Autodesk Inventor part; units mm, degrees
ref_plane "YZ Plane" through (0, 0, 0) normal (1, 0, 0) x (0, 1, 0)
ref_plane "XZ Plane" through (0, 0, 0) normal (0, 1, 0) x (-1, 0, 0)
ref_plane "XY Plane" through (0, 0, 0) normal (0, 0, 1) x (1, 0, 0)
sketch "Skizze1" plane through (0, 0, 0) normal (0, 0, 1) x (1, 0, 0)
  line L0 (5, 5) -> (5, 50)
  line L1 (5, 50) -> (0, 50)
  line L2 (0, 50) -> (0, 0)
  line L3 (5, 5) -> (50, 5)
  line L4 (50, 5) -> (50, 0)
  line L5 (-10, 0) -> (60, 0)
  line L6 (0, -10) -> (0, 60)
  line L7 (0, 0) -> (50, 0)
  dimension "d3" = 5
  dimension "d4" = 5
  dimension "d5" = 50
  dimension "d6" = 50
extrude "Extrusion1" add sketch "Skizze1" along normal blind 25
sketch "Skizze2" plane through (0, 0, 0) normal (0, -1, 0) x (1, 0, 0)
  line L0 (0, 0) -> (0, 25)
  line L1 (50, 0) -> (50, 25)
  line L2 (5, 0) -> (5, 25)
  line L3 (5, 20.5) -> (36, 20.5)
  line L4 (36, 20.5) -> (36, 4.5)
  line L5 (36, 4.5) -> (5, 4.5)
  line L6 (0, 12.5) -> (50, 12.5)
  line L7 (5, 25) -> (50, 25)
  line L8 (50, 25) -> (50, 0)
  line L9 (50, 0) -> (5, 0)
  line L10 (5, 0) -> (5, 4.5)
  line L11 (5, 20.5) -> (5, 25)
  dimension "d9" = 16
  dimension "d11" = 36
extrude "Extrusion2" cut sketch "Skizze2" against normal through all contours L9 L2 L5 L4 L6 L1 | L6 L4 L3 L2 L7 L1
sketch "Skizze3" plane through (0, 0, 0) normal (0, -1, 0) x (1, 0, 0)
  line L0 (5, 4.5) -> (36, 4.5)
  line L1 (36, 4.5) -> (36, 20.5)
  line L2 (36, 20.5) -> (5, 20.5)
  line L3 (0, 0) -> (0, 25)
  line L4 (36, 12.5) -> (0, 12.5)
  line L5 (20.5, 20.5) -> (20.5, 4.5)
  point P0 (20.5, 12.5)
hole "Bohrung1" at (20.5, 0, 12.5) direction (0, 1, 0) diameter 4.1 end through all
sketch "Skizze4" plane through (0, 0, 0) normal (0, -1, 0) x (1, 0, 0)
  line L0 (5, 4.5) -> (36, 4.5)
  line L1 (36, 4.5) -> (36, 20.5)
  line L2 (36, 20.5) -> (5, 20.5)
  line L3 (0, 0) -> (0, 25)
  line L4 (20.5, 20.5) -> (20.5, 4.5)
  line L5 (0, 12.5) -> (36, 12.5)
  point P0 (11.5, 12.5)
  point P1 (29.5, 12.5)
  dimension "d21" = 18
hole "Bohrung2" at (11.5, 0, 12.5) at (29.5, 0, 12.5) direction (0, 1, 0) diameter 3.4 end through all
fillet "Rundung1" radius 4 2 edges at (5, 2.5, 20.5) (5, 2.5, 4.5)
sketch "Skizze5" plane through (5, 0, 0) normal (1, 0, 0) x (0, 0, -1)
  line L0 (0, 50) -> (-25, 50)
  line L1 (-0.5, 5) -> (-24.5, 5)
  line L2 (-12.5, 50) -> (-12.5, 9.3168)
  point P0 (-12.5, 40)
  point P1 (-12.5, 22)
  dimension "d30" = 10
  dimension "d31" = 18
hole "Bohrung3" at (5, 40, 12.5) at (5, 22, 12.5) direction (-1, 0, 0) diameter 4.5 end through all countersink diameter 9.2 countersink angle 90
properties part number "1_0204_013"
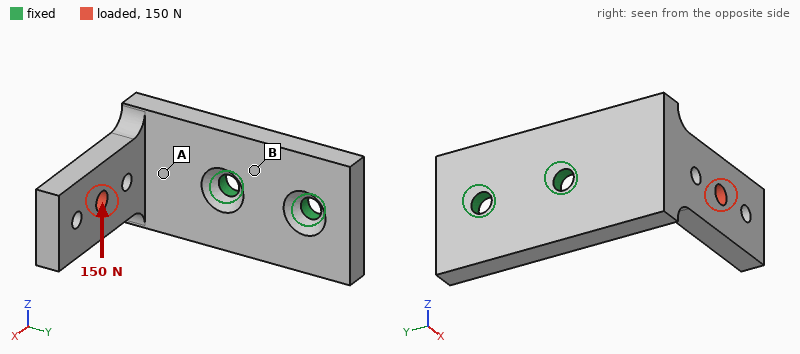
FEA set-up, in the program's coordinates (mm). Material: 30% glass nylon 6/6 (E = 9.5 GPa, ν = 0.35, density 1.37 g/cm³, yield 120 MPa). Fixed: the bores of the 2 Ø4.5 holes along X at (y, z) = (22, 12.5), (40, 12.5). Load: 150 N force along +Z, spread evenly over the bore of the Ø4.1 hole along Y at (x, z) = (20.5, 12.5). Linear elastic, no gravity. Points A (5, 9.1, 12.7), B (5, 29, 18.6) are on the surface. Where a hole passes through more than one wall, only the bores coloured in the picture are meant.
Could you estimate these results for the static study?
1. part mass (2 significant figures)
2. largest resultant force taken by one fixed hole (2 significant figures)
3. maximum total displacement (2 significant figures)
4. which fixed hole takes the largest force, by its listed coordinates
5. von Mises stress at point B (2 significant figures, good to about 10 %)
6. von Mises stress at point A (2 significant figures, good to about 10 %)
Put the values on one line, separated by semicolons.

11 g; 250 N; 0.74 mm; (22, 12.5); 9.2 MPa; 24 MPa
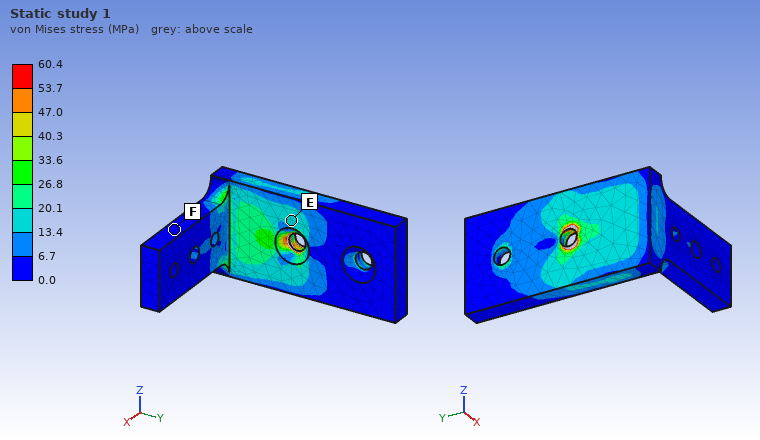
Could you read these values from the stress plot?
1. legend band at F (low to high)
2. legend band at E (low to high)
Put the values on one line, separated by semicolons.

0.0 to 6.7 MPa; 13.4 to 20.1 MPa
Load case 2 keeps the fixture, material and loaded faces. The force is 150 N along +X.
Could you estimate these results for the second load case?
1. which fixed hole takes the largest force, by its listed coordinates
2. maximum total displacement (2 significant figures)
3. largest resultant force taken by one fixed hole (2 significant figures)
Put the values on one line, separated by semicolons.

(22, 12.5); 0.58 mm; 280 N
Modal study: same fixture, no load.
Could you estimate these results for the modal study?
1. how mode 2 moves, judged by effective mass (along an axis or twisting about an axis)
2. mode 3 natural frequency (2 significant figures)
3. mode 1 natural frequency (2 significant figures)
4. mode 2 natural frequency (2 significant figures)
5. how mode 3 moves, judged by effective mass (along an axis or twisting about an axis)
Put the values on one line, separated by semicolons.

along Z; 2900 Hz; 1100 Hz; 1500 Hz; along X
